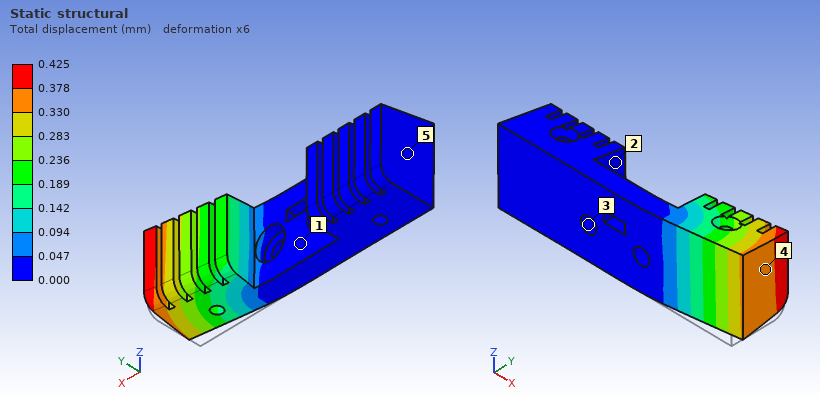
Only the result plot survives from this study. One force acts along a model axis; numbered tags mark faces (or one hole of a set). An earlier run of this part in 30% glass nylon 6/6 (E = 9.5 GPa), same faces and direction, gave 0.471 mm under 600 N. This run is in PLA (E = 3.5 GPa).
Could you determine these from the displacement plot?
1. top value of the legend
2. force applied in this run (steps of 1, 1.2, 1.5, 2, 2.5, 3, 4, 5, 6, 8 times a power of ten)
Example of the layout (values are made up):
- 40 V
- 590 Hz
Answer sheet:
- 0.425 mm
- 200 N
